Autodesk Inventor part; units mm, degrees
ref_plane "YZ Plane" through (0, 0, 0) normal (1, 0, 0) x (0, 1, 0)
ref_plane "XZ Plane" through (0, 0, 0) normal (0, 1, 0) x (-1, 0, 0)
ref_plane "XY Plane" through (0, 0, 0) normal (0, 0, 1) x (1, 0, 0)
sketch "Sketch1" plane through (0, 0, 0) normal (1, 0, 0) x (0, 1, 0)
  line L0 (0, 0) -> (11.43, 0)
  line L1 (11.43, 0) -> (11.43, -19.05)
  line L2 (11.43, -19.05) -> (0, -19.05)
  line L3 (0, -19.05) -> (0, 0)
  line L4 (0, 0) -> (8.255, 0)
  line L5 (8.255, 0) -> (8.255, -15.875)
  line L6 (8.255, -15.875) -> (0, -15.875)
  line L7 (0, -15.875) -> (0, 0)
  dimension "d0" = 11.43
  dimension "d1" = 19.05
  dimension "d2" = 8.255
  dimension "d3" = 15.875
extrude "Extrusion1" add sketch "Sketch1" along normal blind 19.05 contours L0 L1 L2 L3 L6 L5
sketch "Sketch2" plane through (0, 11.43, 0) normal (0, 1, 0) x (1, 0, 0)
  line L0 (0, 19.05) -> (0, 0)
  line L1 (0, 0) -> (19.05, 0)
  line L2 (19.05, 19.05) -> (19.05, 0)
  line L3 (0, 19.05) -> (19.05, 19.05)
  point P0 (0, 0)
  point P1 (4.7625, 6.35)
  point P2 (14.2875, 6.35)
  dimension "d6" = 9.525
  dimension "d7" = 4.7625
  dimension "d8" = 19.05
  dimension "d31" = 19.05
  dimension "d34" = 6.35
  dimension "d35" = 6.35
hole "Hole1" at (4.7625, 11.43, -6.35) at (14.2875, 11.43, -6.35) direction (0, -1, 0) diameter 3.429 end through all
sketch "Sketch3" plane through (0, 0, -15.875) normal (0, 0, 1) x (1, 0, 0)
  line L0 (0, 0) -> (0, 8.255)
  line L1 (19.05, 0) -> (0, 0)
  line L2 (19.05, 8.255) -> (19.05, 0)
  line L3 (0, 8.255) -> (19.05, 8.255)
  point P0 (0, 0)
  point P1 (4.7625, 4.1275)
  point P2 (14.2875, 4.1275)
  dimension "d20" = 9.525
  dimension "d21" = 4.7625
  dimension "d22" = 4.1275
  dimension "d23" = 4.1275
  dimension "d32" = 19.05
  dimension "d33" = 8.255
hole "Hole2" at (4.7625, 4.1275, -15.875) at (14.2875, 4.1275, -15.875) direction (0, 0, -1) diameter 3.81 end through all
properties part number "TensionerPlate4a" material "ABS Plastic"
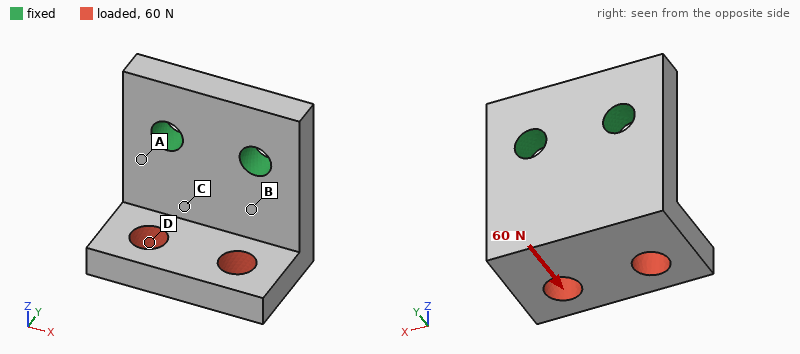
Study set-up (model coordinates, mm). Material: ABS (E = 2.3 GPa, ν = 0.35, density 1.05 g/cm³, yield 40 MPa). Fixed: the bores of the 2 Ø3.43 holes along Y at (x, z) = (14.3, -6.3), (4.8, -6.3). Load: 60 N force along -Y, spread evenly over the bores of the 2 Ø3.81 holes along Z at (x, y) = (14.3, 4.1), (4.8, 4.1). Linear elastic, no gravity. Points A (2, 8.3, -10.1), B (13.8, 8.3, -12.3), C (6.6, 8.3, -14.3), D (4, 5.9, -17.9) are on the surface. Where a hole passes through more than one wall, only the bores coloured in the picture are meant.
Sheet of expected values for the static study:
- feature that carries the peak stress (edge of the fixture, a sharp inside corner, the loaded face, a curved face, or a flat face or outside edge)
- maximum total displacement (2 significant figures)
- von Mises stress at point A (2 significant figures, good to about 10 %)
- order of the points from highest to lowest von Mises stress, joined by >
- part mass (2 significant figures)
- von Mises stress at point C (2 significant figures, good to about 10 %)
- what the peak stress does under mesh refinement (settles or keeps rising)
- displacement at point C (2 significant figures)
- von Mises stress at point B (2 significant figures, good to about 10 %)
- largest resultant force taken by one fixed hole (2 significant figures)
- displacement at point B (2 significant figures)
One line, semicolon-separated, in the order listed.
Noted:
edge of the fixture; 0.35 mm; 12 MPa; A > B > C > D; 1.6 g; 5.4 MPa; keeps rising; 0.12 mm; 8.9 MPa; 30 N; 0.072 mm
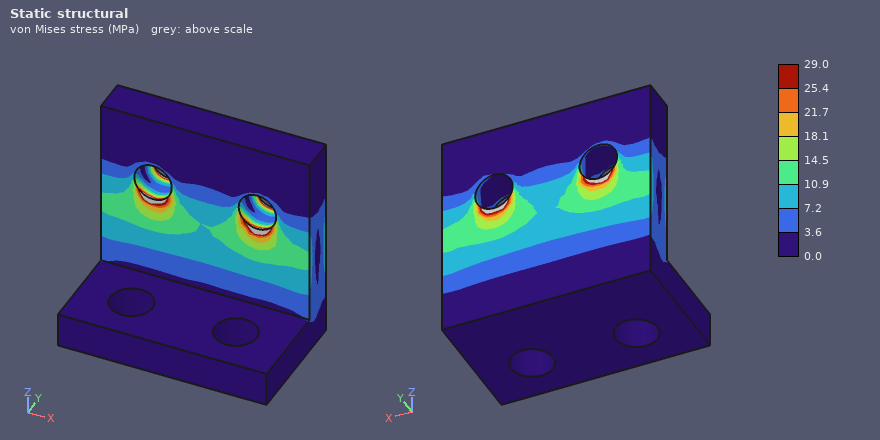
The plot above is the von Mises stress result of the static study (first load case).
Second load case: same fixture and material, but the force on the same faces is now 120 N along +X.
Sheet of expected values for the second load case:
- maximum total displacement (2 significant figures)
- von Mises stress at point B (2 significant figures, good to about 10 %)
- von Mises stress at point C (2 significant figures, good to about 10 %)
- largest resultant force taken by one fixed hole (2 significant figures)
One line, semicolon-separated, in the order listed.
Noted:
0.34 mm; 14 MPa; 16 MPa; 130 N
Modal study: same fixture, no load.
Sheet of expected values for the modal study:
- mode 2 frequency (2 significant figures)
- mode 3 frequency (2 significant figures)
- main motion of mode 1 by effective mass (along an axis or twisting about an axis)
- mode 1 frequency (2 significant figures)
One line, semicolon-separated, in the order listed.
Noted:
4200 Hz; 7100 Hz; along Y; 2600 Hz
